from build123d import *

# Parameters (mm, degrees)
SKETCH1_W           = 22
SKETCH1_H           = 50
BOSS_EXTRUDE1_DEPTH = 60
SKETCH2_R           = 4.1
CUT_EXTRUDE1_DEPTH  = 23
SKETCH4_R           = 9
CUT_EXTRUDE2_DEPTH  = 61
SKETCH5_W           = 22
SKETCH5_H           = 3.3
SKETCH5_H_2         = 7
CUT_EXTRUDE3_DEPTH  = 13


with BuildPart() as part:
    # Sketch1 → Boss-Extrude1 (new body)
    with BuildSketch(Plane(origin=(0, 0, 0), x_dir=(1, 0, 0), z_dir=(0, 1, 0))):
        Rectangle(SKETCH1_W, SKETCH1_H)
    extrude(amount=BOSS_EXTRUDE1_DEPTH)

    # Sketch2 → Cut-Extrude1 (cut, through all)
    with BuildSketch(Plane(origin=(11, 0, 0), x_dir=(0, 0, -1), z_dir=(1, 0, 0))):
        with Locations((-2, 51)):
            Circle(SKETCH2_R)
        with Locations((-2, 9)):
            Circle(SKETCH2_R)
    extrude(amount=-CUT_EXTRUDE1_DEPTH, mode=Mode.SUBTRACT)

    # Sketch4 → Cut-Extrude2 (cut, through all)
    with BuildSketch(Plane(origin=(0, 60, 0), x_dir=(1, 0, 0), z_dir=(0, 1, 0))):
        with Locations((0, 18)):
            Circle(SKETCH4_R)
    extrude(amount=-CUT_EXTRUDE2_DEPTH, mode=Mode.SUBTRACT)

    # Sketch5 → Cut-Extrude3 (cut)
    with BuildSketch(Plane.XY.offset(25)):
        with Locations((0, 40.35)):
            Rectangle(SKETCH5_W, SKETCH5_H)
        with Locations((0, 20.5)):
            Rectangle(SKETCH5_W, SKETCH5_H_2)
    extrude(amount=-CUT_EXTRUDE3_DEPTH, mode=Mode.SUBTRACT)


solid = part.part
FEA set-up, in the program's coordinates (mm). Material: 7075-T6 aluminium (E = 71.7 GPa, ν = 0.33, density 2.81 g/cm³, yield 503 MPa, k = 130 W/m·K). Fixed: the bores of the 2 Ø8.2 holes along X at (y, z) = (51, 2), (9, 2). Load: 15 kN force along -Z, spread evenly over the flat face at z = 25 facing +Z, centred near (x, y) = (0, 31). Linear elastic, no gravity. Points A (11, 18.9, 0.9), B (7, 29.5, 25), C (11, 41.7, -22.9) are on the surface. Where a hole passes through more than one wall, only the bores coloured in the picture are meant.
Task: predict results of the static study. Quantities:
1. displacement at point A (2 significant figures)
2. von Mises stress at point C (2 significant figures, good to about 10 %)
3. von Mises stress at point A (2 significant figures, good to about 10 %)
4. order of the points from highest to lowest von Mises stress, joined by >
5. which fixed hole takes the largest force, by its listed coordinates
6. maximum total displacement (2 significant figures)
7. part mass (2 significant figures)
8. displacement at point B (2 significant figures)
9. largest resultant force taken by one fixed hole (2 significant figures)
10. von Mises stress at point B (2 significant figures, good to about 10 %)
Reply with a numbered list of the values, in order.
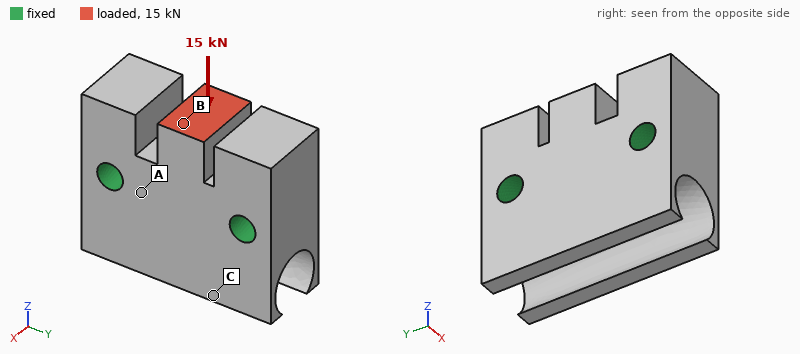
1. 5.8 µm
2. 12 MPa
3. 30 MPa
4. B > A > C
5. (51, 2)
6. 22 µm
7. 130 g
8. 21 µm
9. 8.1 kN
10. 47 MPa
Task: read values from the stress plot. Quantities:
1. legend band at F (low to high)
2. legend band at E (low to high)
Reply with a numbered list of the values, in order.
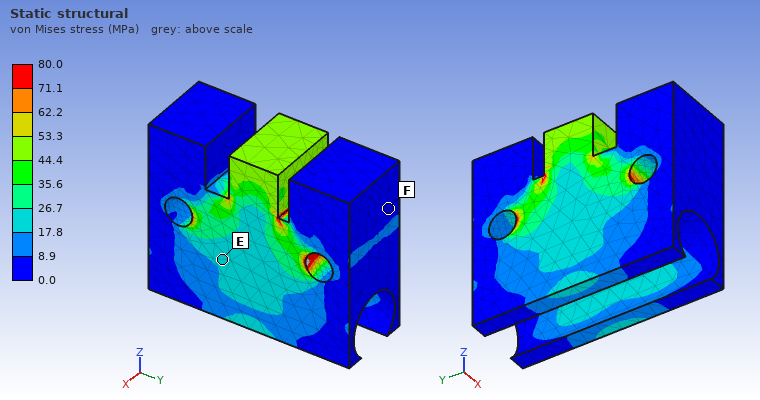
1. 0.0 to 8.9 MPa
2. 17.8 to 26.7 MPa
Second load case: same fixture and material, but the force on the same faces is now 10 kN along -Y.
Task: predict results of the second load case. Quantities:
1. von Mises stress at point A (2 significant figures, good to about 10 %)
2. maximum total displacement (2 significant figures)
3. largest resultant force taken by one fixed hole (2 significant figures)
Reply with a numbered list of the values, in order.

1. 26 MPa
2. 73 µm
3. 8.1 kN
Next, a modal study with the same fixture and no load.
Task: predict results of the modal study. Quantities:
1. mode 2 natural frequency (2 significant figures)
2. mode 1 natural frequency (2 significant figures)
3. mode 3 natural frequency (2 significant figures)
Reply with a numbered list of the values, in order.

1. 9500 Hz
2. 9300 Hz
3. 11 kHz
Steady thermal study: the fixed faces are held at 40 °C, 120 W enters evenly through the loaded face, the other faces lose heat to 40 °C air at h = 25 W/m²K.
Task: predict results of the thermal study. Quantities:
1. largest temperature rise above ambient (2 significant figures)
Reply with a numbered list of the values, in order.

1. 63 K
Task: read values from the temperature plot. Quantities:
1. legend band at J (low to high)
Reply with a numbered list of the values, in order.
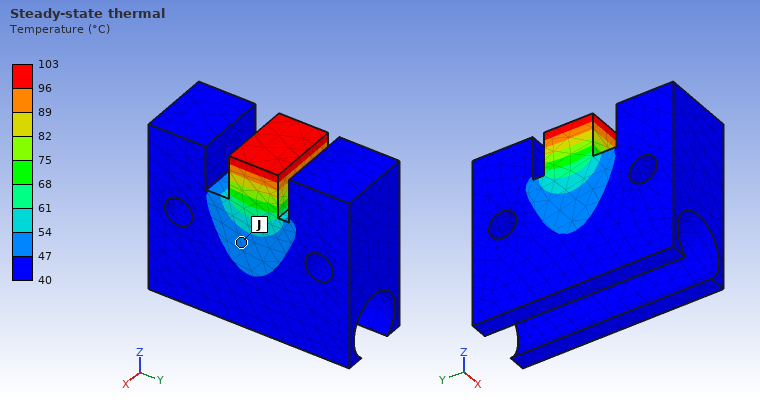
1. 47 to 54 °C
